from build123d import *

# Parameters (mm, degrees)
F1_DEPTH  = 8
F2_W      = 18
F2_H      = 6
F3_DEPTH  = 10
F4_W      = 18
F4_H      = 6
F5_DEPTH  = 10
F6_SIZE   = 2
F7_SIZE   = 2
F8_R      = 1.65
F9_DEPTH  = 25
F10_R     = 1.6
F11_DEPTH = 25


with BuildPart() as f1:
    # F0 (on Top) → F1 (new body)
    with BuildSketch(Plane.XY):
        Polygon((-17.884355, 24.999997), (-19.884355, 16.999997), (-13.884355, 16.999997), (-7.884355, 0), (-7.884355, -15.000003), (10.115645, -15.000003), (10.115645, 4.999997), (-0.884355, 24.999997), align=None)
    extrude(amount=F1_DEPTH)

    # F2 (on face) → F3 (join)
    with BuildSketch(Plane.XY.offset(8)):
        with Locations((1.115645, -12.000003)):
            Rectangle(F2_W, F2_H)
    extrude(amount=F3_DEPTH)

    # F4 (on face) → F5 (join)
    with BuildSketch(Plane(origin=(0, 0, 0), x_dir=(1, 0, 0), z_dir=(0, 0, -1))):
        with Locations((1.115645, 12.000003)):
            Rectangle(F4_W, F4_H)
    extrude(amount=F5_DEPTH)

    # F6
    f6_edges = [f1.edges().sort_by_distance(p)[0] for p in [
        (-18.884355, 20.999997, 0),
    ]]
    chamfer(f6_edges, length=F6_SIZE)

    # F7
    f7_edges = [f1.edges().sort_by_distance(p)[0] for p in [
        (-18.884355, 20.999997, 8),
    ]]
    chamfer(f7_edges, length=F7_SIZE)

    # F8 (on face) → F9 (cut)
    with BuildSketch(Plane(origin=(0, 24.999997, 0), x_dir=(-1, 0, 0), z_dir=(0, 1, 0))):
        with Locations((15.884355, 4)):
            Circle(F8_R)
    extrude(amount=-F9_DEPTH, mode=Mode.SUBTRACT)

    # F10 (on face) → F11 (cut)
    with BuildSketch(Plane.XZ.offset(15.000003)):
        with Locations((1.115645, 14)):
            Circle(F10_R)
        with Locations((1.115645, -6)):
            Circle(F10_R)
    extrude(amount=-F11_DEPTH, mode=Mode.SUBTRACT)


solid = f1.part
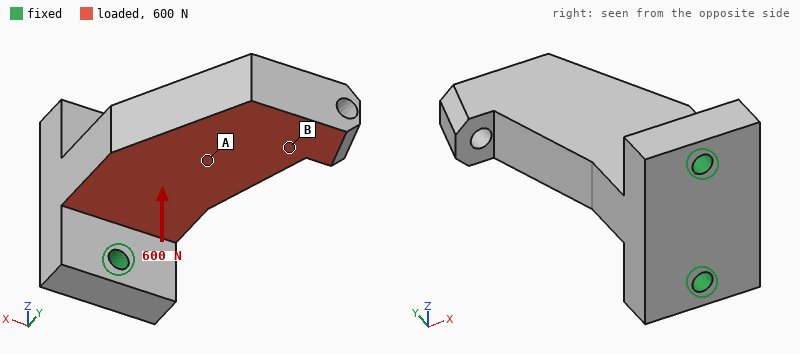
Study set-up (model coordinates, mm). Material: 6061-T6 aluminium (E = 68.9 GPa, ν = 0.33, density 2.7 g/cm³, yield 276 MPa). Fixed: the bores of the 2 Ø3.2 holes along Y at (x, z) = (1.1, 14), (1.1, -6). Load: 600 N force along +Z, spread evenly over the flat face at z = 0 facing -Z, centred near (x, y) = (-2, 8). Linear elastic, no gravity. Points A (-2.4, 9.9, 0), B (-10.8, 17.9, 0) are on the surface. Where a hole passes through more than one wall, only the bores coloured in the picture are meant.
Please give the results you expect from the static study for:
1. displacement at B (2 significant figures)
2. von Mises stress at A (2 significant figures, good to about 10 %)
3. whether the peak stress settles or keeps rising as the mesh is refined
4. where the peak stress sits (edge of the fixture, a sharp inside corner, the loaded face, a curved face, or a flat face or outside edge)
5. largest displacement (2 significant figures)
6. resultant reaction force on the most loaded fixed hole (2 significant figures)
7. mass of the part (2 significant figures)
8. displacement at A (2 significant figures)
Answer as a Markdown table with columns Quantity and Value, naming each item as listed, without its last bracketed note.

| Quantity | Value |
|---|---|
| displacement at B | 0.075 mm |
| von Mises stress at A | 12 MPa |
| whether the peak stress settles or keeps rising as the mesh is refined | keeps rising |
| where the peak stress sits | edge of the fixture |
| largest displacement | 0.10 mm |
| resultant reaction force on the most loaded fixed hole | 770 N |
| mass of the part | 21 g |
| displacement at A | 0.046 mm |
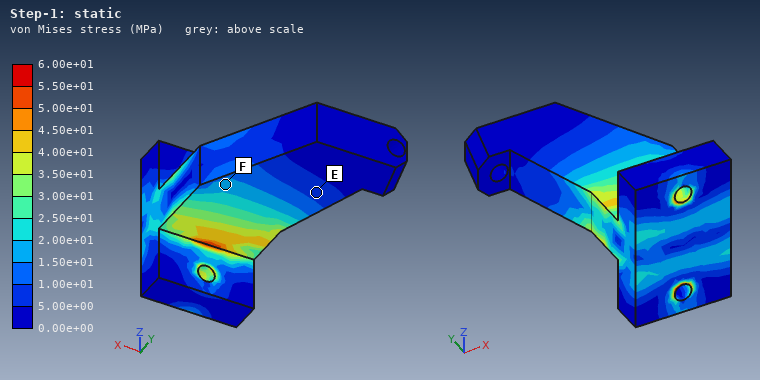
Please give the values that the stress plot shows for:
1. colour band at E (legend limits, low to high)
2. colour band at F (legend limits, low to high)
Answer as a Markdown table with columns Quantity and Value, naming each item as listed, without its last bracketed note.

| Quantity | Value |
|---|---|
| colour band at E | 5.00e+00 to 1.00e+01 MPa |
| colour band at F | 1.50e+01 to 2.00e+01 MPa |
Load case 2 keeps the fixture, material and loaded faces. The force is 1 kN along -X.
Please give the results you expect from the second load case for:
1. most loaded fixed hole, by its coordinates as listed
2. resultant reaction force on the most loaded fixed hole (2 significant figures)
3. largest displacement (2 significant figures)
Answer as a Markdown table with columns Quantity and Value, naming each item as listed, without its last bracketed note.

| Quantity | Value |
|---|---|
| most loaded fixed hole, by its coordinates as listed | (1.1, -6) |
| resultant reaction force on the most loaded fixed hole | 690 N |
| largest displacement | 0.15 mm |
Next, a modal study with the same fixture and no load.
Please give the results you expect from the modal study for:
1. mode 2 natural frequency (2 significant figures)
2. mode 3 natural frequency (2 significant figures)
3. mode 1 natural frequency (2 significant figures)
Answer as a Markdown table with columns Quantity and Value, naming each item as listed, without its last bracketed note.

| Quantity | Value |
|---|---|
| mode 2 natural frequency | 4400 Hz |
| mode 3 natural frequency | 14 kHz |
| mode 1 natural frequency | 4200 Hz |
